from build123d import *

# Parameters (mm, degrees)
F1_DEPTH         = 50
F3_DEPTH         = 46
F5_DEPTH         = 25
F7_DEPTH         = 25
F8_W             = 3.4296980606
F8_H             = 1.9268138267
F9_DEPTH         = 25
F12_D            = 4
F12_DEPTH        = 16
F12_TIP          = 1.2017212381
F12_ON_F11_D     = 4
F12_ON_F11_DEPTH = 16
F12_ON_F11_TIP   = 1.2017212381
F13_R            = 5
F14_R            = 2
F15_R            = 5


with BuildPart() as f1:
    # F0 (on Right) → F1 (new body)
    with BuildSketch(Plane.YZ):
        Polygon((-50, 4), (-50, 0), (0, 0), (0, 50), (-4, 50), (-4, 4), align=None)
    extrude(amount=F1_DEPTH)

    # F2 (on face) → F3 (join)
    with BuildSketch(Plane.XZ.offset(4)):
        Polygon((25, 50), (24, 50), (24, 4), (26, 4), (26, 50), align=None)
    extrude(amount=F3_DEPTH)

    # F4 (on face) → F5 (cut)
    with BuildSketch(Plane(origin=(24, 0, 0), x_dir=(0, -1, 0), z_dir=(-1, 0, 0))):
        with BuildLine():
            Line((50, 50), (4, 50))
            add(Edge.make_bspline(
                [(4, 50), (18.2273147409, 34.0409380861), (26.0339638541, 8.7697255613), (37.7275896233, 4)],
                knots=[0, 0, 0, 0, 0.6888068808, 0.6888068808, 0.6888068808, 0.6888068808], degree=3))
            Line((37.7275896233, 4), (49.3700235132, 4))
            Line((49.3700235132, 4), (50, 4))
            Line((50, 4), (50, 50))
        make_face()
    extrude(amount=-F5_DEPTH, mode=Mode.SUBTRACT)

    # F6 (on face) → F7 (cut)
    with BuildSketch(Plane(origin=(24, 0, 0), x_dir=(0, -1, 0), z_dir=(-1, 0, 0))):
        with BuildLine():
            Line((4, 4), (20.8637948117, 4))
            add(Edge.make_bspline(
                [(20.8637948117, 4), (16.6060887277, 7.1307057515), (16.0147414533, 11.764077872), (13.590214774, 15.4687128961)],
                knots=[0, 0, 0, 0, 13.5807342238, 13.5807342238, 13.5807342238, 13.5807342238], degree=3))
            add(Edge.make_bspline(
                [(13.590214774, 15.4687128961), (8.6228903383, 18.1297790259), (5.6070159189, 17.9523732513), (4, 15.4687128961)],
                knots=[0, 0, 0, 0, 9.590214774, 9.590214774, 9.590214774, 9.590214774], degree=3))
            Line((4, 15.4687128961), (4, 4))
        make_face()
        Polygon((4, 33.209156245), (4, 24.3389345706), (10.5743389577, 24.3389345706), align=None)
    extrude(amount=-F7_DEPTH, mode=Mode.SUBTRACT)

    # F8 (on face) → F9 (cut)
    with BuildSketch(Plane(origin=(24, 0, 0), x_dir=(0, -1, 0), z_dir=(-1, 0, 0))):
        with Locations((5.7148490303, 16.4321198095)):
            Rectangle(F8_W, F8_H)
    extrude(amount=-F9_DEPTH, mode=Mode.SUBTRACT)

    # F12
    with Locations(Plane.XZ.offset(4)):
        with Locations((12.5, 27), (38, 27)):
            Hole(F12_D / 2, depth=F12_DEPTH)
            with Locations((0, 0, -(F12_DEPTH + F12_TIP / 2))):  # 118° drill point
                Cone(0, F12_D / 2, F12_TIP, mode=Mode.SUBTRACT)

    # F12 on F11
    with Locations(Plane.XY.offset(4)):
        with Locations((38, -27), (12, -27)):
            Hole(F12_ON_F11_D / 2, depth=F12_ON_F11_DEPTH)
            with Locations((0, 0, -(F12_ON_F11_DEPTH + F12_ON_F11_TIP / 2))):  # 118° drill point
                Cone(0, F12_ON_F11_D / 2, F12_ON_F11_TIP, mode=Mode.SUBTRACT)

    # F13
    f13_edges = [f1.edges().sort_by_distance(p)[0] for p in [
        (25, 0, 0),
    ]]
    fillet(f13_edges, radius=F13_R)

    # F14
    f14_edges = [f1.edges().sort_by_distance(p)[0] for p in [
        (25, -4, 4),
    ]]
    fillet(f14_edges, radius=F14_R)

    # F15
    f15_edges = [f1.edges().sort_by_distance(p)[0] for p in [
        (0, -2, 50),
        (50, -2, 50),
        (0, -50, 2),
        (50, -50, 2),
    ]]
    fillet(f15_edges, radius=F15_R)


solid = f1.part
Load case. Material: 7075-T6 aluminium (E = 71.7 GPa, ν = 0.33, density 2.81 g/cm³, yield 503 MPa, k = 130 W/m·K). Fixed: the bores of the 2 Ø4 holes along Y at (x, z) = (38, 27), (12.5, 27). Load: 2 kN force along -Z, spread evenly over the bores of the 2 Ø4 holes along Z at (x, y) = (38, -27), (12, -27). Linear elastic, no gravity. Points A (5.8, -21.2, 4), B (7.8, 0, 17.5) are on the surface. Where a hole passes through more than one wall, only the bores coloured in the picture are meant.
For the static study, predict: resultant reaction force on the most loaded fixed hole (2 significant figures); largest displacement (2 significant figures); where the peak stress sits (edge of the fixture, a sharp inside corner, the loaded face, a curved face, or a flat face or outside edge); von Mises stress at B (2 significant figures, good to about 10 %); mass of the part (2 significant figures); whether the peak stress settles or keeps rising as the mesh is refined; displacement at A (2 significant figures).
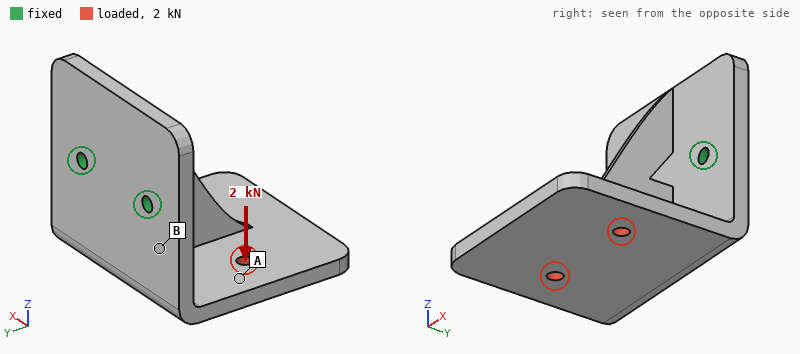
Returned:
1.0 kN
0.87 mm
edge of the fixture
110 MPa
55 g
keeps rising
0.47 mm
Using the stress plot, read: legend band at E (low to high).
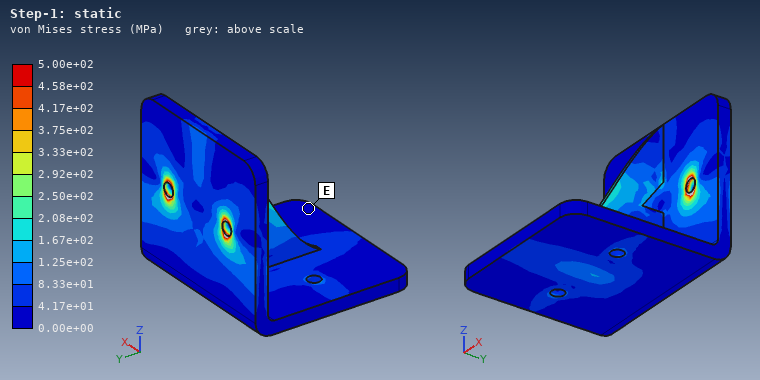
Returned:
0.00e+00 to 4.17e+01 MPa
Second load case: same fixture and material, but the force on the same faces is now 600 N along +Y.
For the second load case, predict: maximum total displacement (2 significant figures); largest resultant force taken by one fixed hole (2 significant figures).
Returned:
0.22 mm
310 N
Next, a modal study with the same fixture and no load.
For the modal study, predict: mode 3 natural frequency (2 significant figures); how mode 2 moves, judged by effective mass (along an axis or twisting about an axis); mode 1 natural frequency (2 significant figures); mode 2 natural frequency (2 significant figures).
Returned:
3200 Hz
along X
1500 Hz
1500 Hz
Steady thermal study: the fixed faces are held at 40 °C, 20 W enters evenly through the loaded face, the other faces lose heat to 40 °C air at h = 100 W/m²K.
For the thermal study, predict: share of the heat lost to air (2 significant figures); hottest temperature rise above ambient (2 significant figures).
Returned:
54 %
23 K
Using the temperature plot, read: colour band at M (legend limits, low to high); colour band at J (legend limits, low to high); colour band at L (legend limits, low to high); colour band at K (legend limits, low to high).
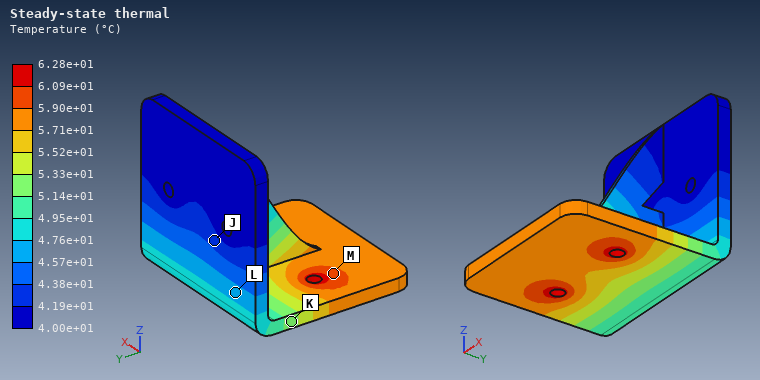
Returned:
5.90e+01 to 6.09e+01 °C
4.19e+01 to 4.38e+01 °C
4.57e+01 to 4.76e+01 °C
5.14e+01 to 5.33e+01 °C
